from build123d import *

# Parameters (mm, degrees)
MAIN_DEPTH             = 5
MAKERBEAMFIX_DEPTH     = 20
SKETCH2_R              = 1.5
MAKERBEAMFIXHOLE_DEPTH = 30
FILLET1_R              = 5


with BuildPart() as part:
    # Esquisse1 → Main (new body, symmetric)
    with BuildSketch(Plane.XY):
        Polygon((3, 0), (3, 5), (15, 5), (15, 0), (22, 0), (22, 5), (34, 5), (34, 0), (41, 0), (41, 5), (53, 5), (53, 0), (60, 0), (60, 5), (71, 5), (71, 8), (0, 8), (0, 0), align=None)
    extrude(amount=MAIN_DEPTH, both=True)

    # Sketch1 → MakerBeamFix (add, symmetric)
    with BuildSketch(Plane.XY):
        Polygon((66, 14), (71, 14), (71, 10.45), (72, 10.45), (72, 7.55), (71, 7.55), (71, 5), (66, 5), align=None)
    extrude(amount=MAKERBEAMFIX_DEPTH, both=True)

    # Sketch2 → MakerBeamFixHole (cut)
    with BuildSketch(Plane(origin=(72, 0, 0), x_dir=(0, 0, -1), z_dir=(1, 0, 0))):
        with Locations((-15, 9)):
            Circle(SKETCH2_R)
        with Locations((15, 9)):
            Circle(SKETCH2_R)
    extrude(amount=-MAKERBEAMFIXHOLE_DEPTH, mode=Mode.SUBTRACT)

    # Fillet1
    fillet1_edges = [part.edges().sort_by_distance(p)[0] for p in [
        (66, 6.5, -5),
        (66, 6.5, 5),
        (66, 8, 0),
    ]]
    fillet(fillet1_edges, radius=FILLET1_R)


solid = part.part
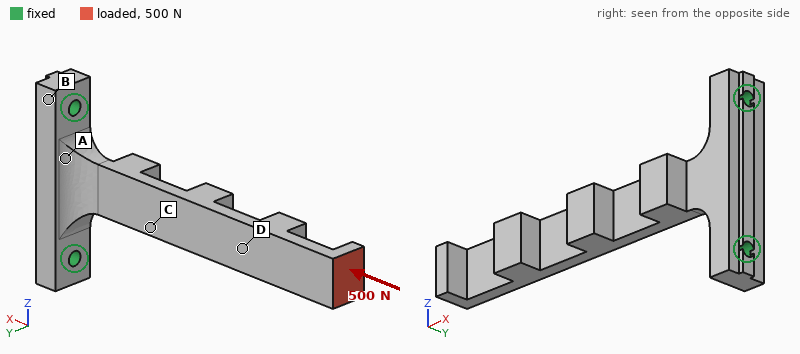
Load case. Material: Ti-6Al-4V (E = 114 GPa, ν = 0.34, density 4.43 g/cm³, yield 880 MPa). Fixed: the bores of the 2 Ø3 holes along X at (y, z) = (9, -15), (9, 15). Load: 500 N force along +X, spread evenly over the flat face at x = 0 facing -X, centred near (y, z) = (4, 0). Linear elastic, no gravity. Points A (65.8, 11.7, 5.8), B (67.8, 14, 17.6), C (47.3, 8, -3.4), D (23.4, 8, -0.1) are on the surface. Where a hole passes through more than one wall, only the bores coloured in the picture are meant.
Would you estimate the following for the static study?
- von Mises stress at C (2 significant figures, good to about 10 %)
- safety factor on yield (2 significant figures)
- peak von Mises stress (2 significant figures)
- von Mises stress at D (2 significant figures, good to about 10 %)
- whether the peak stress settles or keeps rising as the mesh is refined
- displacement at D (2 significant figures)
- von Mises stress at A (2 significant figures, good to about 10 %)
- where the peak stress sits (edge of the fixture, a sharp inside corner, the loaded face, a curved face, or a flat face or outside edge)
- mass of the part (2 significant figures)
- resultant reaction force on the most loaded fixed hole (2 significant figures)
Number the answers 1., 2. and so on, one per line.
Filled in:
1. 66 MPa
2. 7.5
3. 120 MPa
4. 58 MPa
5. settles
6. 0.35 mm
7. 21 MPa
8. a curved face
9. 23 g
10. 280 N
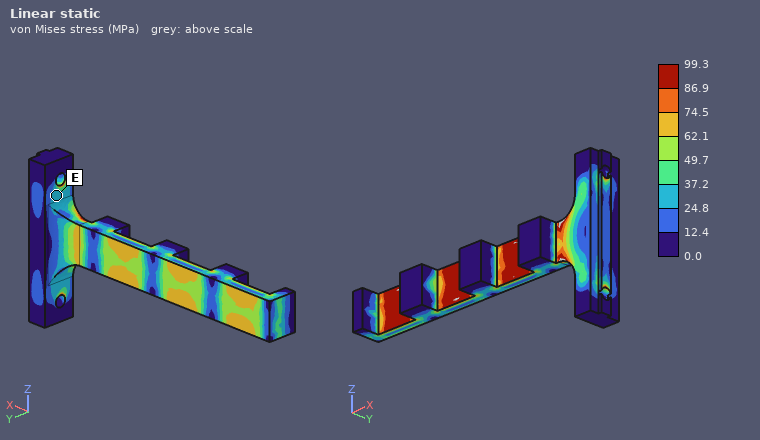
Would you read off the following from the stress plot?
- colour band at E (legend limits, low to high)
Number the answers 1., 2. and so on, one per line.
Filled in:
1. 24.8 to 37.2 MPa
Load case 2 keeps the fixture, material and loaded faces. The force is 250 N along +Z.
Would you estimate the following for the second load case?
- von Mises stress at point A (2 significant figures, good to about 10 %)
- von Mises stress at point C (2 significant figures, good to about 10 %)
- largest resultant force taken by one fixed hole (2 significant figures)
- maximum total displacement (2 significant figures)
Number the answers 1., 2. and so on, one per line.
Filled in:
1. 40 MPa
2. 160 MPa
3. 790 N
4. 0.86 mm
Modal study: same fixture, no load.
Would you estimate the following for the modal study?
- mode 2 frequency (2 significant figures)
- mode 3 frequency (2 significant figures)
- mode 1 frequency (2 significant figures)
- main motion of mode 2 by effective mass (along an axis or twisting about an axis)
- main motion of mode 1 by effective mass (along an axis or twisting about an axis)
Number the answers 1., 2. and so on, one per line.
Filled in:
1. 1500 Hz
2. 3000 Hz
3. 510 Hz
4. along Z
5. along Y
